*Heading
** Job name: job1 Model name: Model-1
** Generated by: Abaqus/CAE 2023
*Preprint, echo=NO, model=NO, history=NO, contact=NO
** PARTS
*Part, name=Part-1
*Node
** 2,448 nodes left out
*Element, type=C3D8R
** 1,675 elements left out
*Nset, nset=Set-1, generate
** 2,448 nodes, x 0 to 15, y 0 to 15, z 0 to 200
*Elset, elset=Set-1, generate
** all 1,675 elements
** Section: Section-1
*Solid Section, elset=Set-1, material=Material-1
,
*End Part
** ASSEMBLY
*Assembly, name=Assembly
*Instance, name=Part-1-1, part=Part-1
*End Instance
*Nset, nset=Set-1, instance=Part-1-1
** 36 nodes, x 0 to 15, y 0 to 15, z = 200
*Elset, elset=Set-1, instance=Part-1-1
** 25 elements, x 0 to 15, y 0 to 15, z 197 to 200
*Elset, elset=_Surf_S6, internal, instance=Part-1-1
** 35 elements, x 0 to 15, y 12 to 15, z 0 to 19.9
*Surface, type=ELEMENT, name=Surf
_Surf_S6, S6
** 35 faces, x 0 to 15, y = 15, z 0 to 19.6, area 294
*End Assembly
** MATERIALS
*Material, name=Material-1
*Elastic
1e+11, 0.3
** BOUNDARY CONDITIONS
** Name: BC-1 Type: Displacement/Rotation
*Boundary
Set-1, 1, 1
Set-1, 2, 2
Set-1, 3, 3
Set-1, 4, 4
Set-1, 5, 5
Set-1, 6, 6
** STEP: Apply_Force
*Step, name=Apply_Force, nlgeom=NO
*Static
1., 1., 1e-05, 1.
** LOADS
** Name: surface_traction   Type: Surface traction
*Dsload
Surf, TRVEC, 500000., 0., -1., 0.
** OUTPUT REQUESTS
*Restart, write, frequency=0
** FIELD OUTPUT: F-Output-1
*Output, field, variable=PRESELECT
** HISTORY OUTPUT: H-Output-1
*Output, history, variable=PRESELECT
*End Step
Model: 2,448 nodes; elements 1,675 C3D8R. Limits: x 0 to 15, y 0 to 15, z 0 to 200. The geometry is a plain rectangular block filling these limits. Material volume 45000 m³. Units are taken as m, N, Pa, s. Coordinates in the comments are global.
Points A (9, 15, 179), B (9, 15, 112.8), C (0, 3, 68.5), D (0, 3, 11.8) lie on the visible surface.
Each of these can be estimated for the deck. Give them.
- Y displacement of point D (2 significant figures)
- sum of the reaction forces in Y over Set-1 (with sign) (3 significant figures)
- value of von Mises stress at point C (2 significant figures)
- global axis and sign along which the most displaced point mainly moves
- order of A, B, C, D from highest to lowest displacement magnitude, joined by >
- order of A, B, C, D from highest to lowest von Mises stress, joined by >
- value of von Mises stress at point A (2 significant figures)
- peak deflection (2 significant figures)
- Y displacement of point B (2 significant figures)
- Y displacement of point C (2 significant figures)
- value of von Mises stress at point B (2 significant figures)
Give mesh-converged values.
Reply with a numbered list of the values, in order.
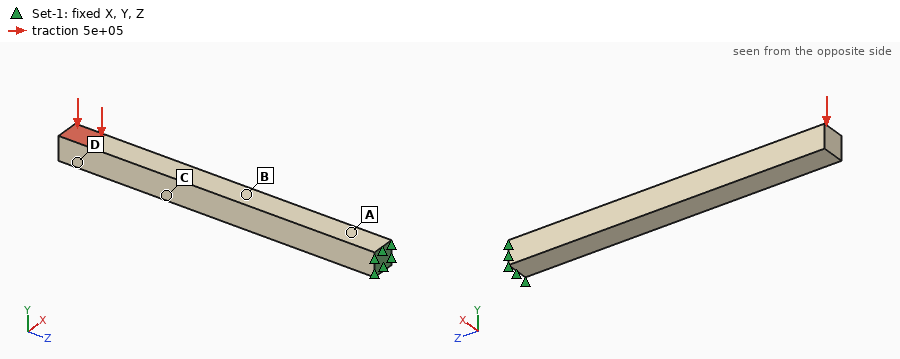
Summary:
1. -0.79 m
2. 1.47e+08 N
3. 9.3e+06 Pa
4. -Y
5. D > C > B > A
6. A > B > C > D
7. 4.4e+07 Pa
8. 0.86 m
9. -0.21 m
10. -0.44 m
11. 2.7e+07 Pa
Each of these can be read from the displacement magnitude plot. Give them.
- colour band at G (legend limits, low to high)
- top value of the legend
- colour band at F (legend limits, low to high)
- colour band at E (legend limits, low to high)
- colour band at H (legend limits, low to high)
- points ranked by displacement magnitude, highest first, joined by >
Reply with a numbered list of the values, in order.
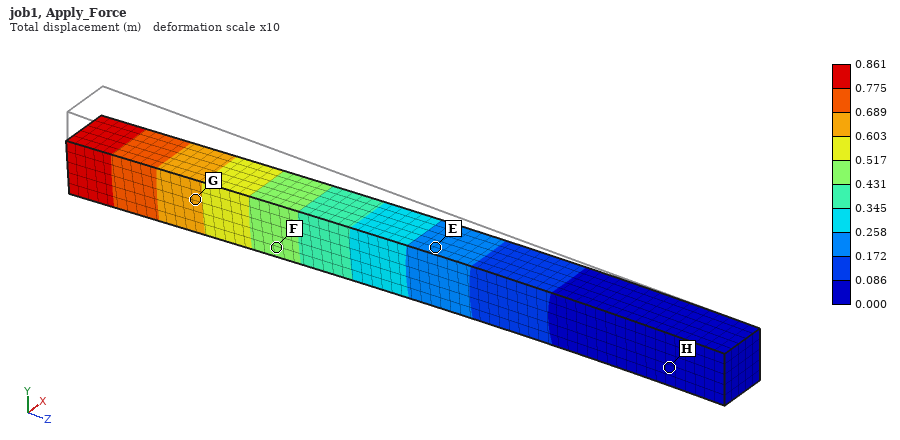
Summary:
1. 0.603 to 0.689 m
2. 0.861 m
3. 0.431 to 0.517 m
4. 0.172 to 0.258 m
5. 0.000 to 0.086 m
6. G > F > E > H
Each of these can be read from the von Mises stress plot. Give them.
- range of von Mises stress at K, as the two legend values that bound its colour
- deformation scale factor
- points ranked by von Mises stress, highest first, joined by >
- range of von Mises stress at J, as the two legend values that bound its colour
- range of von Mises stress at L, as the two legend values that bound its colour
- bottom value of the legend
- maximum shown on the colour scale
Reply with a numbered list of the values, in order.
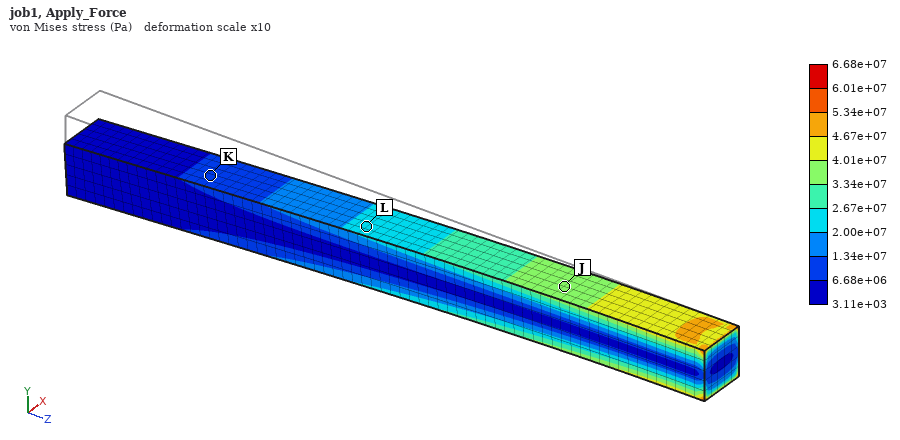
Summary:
1. 6.68e+06 to 1.34e+07 Pa
2. 10
3. J > L > K
4. 3.34e+07 to 4.01e+07 Pa
5. 2.00e+07 to 2.67e+07 Pa
6. 3.11e+03 Pa
7. 6.68e+07 Pa
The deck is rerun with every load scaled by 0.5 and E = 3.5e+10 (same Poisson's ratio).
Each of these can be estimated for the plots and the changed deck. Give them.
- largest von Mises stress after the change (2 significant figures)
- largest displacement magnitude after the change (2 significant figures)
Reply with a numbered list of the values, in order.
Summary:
1. 3.3e+07 Pa
2. 1.2 m
